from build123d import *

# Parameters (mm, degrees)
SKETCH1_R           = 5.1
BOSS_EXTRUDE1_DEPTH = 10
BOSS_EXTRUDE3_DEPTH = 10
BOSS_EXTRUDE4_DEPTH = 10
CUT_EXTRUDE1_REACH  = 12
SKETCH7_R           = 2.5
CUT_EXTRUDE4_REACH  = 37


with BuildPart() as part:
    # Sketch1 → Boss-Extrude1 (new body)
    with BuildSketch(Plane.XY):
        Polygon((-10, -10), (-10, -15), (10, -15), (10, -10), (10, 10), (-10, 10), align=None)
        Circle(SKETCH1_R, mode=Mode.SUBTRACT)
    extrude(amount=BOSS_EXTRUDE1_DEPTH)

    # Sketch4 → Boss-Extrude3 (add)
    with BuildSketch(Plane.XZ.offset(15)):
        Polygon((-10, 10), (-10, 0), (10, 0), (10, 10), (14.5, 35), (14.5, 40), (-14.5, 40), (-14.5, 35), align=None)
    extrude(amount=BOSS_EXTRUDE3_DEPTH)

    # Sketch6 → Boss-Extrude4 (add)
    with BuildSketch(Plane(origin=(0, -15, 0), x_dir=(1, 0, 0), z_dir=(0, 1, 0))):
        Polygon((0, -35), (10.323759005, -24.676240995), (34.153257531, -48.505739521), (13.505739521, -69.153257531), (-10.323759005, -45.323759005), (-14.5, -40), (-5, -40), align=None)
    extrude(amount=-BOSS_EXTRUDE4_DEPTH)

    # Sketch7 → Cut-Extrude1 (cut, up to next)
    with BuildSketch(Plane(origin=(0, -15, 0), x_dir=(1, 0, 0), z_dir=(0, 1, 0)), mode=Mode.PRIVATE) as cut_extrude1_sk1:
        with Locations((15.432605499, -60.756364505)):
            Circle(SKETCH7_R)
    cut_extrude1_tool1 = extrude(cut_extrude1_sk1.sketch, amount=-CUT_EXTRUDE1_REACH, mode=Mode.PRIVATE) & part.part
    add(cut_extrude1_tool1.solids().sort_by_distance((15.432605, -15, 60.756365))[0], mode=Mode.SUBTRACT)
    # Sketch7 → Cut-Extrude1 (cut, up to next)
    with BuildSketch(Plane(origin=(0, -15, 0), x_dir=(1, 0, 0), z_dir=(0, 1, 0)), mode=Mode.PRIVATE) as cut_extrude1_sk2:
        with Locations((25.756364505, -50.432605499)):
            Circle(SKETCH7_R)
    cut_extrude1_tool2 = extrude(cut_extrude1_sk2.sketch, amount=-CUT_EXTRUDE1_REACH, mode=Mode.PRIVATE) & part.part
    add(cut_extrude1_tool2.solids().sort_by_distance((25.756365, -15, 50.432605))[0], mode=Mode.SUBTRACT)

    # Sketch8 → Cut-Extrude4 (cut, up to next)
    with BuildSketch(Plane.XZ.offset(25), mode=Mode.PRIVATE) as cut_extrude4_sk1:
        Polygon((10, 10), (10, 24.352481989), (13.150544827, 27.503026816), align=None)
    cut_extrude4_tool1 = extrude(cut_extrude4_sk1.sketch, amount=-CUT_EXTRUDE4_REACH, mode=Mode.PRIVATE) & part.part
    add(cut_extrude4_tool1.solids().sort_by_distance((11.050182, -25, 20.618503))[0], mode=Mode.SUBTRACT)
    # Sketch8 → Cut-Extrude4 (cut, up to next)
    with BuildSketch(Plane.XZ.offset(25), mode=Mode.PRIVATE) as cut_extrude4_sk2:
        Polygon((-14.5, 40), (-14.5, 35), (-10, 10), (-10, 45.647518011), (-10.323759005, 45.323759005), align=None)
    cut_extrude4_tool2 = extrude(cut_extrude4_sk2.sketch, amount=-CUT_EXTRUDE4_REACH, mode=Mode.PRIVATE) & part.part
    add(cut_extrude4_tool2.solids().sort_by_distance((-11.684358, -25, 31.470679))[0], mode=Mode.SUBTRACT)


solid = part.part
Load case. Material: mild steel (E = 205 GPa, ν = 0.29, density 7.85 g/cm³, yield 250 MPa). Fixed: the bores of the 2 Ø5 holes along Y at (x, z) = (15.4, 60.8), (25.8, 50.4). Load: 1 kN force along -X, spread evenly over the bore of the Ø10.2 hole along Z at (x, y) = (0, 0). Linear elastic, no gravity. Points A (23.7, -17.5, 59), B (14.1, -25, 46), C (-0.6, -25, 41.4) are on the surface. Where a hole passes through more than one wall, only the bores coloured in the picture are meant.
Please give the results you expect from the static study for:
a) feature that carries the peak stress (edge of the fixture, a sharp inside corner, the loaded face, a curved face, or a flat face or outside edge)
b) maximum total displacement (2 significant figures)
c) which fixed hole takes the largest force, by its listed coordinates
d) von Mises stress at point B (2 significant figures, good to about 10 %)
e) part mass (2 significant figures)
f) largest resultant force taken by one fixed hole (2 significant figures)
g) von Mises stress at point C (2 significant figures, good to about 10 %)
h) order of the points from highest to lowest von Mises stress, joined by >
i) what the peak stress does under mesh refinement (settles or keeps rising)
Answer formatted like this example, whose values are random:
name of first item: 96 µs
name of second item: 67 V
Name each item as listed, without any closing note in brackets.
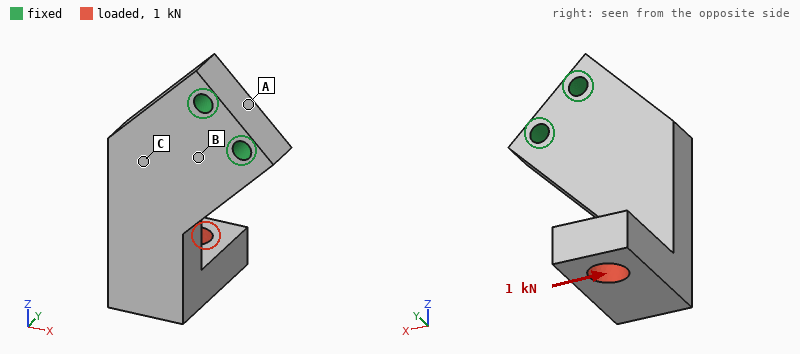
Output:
feature that carries the peak stress: edge of the fixture
maximum total displacement: 0.10 mm
which fixed hole takes the largest force, by its listed coordinates: (25.8, 50.4)
von Mises stress at point B: 27 MPa
part mass: 160 g
largest resultant force taken by one fixed hole: 3.2 kN
von Mises stress at point C: 42 MPa
order of the points from highest to lowest von Mises stress, joined by >: C > B > A
what the peak stress does under mesh refinement: keeps rising
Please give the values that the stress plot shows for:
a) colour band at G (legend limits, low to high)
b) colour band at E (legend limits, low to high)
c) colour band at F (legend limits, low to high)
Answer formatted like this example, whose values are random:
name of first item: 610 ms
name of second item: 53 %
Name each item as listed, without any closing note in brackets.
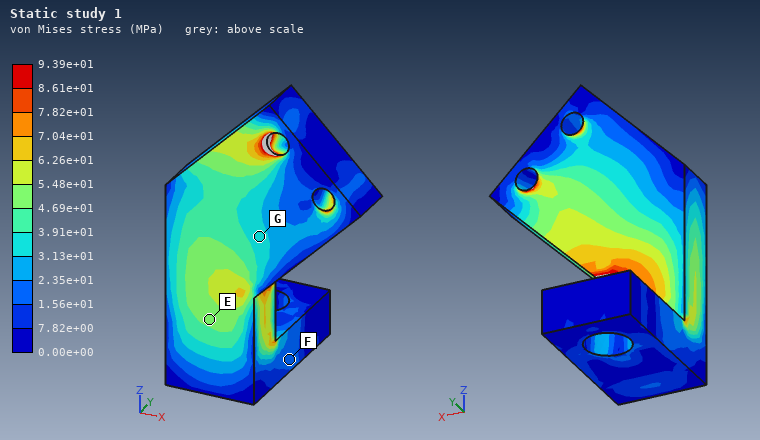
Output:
colour band at G: 3.13e+01 to 3.91e+01 MPa
colour band at E: 4.69e+01 to 5.48e+01 MPa
colour band at F: 1.56e+01 to 2.35e+01 MPa
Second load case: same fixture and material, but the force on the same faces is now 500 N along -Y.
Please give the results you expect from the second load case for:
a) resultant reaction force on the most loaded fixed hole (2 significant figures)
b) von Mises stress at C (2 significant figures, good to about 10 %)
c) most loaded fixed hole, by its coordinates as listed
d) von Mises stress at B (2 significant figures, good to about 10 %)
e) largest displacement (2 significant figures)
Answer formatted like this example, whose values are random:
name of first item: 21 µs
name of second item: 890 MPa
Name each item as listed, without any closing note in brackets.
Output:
resultant reaction force on the most loaded fixed hole: 680 N
von Mises stress at C: 32 MPa
most loaded fixed hole, by its coordinates as listed: (25.8, 50.4)
von Mises stress at B: 42 MPa
largest displacement: 88 µm
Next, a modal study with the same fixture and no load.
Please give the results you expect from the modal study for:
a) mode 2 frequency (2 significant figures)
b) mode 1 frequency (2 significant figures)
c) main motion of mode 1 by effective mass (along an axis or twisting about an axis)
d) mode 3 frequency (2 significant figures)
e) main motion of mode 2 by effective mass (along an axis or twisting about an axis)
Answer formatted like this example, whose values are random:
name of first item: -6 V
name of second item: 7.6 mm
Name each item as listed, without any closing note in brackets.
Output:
mode 2 frequency: 3200 Hz
mode 1 frequency: 1700 Hz
main motion of mode 1 by effective mass: along Y
mode 3 frequency: 5700 Hz
main motion of mode 2 by effective mass: along X
